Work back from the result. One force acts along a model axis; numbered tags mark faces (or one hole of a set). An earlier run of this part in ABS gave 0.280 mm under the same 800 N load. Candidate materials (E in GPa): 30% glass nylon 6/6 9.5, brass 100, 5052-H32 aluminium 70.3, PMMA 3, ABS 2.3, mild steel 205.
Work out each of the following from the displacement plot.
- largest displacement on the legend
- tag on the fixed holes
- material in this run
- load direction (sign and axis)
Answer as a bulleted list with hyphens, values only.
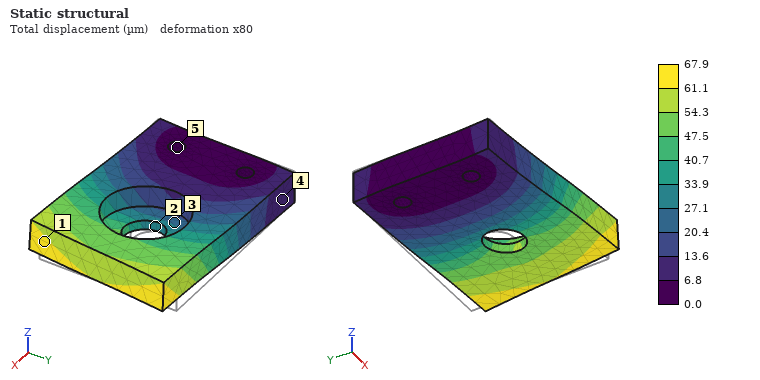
- 67.9 µm
- 5
- 30% glass nylon 6/6
- -Y
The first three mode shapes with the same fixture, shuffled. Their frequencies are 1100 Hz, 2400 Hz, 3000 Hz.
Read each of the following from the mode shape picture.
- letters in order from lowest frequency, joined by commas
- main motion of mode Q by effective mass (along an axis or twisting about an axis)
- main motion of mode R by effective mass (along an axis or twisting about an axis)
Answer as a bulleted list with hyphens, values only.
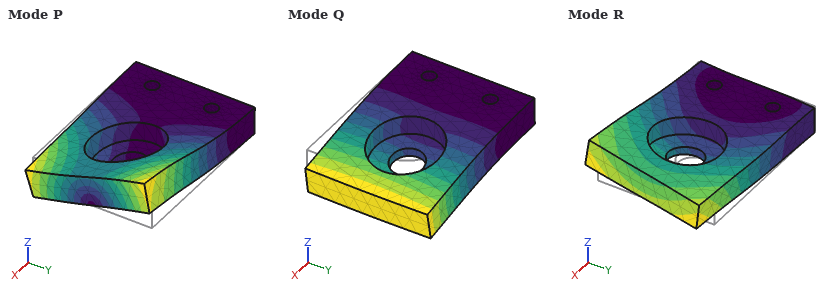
- Q, P, R
- along Z
- along Y
